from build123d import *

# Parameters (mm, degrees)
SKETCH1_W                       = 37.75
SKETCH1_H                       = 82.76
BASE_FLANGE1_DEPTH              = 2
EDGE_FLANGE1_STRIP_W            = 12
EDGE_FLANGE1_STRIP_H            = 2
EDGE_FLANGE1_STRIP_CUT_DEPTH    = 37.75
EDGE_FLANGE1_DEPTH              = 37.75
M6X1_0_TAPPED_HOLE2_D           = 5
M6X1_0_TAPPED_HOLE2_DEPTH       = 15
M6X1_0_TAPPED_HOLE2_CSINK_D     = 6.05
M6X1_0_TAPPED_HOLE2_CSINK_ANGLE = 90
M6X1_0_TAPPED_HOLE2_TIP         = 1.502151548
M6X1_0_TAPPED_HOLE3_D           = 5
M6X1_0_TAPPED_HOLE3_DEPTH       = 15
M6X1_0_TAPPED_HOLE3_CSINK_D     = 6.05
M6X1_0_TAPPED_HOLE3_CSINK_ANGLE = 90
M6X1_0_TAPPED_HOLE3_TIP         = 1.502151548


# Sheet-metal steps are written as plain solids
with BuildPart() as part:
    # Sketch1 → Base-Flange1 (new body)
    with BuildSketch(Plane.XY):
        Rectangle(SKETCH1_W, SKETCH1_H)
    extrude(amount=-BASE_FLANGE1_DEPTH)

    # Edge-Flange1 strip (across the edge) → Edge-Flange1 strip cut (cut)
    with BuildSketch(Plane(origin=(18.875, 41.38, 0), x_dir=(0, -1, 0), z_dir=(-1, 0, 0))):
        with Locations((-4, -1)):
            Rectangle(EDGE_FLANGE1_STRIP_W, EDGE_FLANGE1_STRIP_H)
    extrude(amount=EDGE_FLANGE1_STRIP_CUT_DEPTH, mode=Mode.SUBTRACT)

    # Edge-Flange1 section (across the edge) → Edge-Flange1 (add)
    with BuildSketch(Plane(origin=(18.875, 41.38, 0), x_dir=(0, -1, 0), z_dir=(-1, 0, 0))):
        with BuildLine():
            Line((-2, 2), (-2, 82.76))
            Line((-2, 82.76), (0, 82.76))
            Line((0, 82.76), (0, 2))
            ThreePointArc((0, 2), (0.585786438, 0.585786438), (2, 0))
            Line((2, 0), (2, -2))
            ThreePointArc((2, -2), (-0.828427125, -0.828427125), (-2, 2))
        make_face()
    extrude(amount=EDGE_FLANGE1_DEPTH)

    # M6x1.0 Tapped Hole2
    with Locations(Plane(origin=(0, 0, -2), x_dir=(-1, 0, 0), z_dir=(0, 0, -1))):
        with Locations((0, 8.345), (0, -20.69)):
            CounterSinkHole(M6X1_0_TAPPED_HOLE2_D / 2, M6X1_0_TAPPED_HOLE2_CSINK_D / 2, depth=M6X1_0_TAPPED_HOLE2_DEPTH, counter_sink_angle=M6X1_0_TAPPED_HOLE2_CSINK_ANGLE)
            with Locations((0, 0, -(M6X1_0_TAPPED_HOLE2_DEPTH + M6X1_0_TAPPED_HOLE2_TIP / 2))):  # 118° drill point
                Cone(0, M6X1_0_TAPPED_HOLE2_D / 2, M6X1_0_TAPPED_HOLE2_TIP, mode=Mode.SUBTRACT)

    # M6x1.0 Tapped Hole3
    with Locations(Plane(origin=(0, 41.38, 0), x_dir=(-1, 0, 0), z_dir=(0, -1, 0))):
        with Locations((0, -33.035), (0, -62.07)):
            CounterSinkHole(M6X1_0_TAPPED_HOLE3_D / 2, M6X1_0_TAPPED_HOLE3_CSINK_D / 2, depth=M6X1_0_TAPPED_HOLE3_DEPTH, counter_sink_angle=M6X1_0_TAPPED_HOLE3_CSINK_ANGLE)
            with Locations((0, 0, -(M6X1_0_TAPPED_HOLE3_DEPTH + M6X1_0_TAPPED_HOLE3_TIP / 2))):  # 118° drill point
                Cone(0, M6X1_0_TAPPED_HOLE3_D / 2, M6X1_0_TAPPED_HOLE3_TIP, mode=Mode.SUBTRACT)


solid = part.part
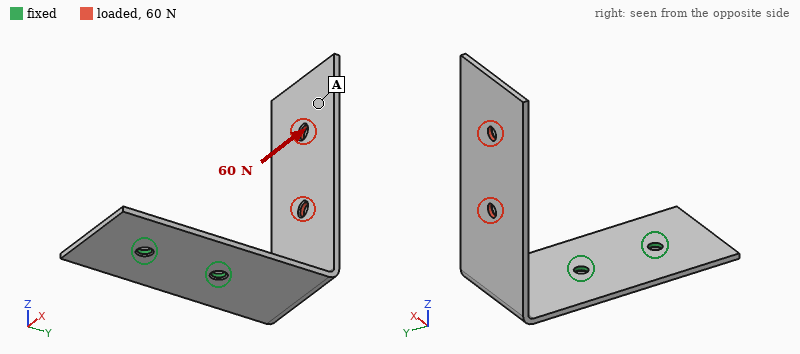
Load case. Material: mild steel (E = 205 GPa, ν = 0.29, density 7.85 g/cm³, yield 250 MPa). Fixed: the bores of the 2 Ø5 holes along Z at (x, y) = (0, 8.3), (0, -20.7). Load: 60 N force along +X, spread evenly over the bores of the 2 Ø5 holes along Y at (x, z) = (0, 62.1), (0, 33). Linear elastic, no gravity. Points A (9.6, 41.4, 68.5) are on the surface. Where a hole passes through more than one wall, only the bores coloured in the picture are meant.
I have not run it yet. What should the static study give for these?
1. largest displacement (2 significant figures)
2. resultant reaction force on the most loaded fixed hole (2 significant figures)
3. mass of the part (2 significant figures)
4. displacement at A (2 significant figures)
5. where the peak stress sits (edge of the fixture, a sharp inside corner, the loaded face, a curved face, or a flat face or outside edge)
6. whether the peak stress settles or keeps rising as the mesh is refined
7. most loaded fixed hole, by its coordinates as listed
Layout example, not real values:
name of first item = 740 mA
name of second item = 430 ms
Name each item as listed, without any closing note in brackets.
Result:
largest displacement = 0.98 mm
resultant reaction force on the most loaded fixed hole = 120 N
mass of the part = 97 g
displacement at A = 0.80 mm
where the peak stress sits = edge of the fixture
whether the peak stress settles or keeps rising as the mesh is refined = keeps rising
most loaded fixed hole, by its coordinates as listed = (0, 8.3)
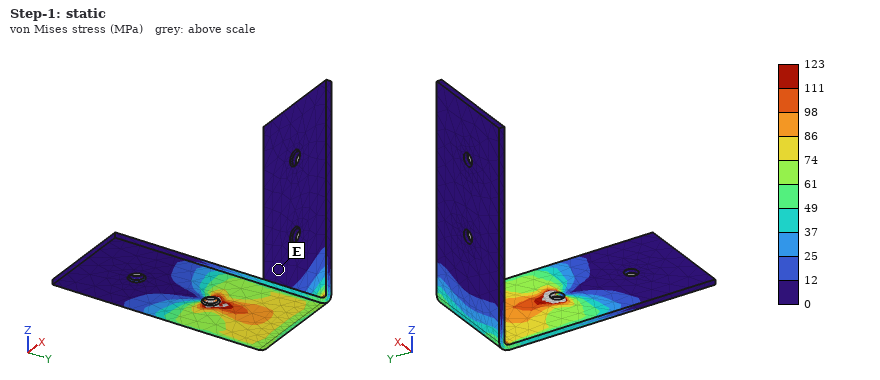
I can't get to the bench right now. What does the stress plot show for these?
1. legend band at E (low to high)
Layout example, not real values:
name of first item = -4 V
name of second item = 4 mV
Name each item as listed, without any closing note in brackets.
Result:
legend band at E = 0 to 12 MPa
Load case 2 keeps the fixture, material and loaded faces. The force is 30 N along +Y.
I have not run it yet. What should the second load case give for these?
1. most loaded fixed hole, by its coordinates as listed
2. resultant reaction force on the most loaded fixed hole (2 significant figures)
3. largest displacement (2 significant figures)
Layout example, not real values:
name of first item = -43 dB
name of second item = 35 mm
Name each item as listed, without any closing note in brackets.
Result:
most loaded fixed hole, by its coordinates as listed = (0, 8.3)
resultant reaction force on the most loaded fixed hole = 45 N
largest displacement = 1.2 mm
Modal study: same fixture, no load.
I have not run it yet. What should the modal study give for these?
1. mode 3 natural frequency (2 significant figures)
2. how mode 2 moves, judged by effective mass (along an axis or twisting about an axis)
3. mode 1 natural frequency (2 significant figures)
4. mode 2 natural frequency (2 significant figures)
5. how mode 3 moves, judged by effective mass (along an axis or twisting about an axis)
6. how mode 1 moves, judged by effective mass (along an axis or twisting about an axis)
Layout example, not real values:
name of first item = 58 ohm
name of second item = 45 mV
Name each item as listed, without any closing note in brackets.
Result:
mode 3 natural frequency = 580 Hz
how mode 2 moves, judged by effective mass = along X
mode 1 natural frequency = 140 Hz
mode 2 natural frequency = 230 Hz
how mode 3 moves, judged by effective mass = along Z
how mode 1 moves, judged by effective mass = along Y
